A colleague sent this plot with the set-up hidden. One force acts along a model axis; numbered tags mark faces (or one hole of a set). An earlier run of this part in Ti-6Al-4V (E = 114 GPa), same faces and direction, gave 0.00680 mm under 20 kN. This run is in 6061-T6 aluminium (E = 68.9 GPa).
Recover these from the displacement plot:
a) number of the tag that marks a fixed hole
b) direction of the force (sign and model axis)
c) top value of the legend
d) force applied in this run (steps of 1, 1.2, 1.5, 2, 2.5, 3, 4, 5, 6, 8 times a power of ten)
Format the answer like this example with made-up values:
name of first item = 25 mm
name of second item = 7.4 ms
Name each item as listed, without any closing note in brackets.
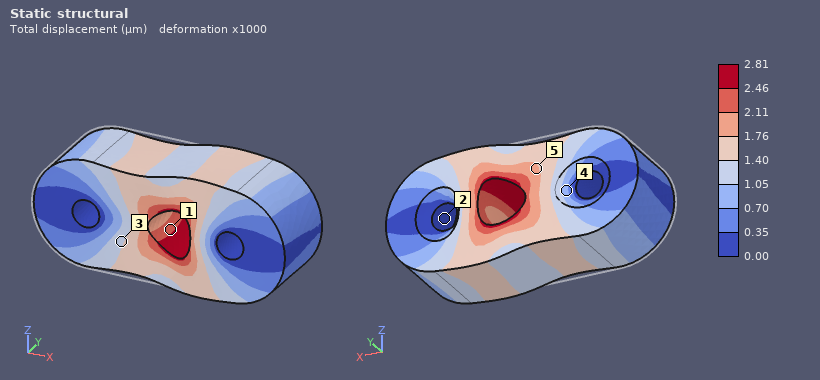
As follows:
number of the tag that marks a fixed hole = 2
direction of the force = +X
top value of the legend = 2.81 µm
force applied in this run = 5 kN
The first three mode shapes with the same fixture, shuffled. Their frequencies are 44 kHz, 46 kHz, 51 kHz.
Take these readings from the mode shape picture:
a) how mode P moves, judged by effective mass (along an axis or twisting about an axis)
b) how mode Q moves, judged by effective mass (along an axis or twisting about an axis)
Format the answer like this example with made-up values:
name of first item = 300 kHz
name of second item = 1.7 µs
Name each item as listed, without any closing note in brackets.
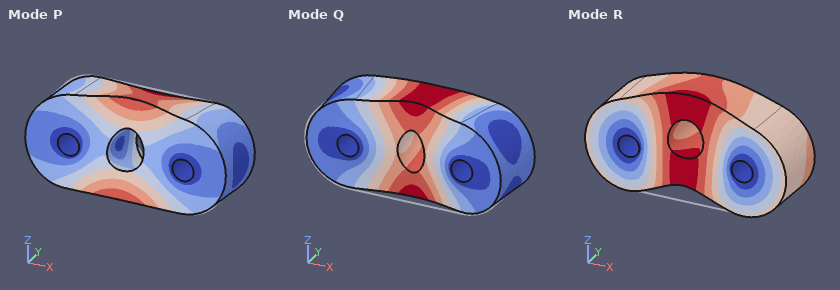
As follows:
how mode P moves, judged by effective mass = twisting about X
how mode Q moves, judged by effective mass = along Y
